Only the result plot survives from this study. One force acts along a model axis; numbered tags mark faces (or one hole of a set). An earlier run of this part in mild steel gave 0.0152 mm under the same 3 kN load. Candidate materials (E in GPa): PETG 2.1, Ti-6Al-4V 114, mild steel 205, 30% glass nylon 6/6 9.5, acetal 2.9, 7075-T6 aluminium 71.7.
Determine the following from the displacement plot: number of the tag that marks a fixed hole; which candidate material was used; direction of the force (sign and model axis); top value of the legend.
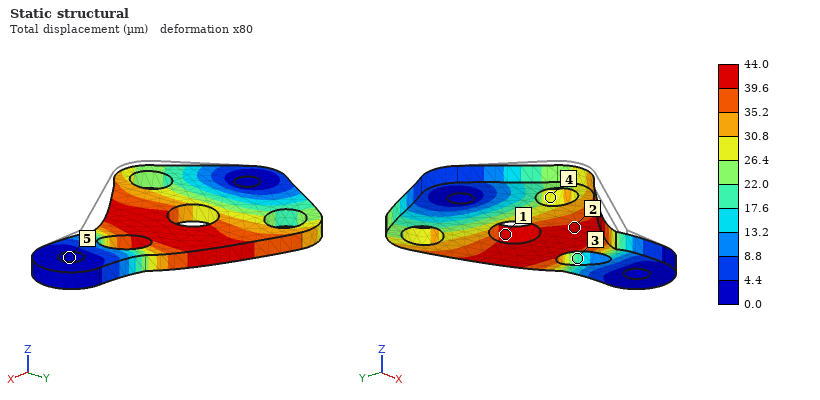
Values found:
5
7075-T6 aluminium
+Y
44.0 µm
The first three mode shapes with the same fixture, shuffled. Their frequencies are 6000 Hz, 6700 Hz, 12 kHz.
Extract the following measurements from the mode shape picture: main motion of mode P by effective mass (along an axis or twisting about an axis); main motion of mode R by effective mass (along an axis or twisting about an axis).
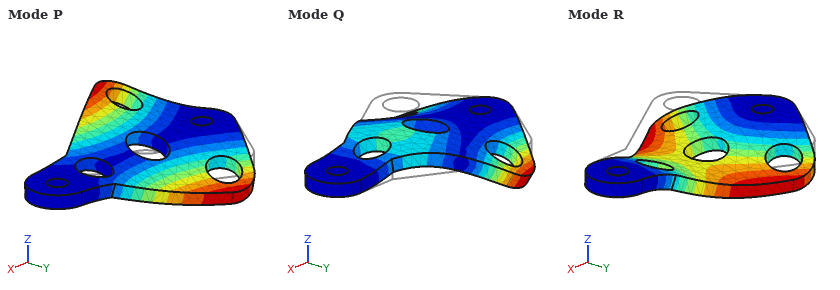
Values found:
twisting about X
along Z
